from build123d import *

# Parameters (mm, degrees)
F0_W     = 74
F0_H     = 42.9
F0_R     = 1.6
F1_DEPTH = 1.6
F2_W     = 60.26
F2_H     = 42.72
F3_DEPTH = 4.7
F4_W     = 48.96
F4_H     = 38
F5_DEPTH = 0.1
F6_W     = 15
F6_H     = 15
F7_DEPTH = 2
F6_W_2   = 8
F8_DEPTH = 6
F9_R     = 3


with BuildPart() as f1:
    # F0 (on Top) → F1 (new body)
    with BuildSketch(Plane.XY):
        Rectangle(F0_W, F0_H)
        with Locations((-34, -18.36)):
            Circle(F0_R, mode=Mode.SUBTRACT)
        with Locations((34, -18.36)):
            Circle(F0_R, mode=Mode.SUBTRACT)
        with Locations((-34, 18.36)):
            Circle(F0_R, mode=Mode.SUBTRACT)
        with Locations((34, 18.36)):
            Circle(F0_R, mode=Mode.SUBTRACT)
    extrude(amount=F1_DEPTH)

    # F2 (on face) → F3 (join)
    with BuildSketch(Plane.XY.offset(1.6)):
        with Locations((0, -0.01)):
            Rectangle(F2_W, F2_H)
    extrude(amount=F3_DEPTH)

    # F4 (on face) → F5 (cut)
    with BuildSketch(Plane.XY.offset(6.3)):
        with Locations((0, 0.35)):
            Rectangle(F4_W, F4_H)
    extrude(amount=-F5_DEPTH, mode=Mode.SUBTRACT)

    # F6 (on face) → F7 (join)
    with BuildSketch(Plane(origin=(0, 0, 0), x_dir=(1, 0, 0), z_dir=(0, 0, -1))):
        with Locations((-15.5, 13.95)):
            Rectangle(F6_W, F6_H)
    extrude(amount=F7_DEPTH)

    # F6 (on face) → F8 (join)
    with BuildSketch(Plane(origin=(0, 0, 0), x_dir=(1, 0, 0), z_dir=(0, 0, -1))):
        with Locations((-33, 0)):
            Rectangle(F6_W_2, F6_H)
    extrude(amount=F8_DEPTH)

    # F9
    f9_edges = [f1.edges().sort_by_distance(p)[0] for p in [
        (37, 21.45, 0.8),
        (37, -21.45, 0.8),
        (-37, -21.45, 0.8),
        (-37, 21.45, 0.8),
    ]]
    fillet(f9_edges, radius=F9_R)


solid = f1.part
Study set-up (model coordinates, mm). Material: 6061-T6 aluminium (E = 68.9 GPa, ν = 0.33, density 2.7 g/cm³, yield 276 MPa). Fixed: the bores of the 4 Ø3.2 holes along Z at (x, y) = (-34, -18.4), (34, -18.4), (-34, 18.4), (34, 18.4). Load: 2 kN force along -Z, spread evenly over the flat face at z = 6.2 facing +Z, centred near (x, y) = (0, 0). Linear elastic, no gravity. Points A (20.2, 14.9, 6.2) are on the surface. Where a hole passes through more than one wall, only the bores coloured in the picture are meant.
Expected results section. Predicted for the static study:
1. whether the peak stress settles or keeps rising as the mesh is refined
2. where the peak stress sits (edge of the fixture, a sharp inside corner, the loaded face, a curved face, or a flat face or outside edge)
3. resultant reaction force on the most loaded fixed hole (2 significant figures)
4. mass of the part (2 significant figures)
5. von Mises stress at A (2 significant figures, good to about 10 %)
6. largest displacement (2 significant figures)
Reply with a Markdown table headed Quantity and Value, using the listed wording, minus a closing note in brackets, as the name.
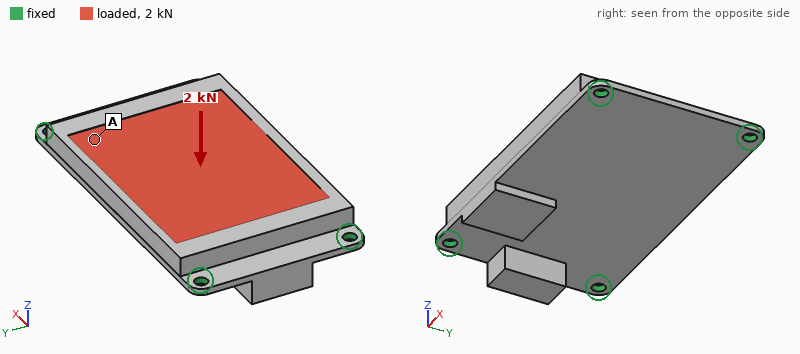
| Quantity | Value |
|---|---|
| whether the peak stress settles or keeps rising as the mesh is refined | keeps rising |
| where the peak stress sits | edge of the fixture |
| resultant reaction force on the most loaded fixed hole | 1.2 kN |
| mass of the part | 49 g |
| von Mises stress at A | 35 MPa |
| largest displacement | 0.11 mm |
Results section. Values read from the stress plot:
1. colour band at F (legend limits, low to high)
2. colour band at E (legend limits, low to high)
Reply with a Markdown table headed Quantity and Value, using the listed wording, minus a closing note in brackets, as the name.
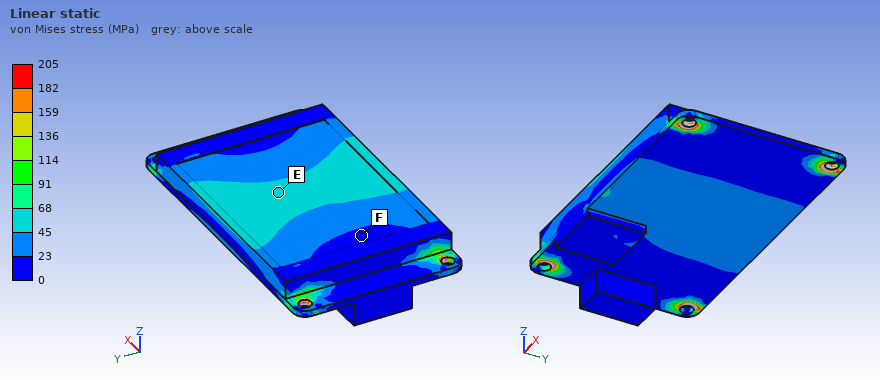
| Quantity | Value |
|---|---|
| colour band at F | 0 to 23 MPa |
| colour band at E | 45 to 68 MPa |
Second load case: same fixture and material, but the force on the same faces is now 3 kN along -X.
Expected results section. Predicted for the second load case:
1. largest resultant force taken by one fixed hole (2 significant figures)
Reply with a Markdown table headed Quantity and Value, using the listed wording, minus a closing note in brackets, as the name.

| Quantity | Value |
|---|---|
| largest resultant force taken by one fixed hole | 810 N |
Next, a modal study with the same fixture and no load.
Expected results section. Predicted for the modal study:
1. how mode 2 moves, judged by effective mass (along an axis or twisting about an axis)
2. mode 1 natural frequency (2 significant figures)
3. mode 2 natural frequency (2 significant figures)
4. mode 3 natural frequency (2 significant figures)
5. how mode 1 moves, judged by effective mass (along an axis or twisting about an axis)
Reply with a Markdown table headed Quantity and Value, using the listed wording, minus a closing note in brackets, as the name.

| Quantity | Value |
|---|---|
| how mode 2 moves, judged by effective mass | twisting about X |
| mode 1 natural frequency | 3900 Hz |
| mode 2 natural frequency | 6700 Hz |
| mode 3 natural frequency | 8500 Hz |
| how mode 1 moves, judged by effective mass | along Z |
